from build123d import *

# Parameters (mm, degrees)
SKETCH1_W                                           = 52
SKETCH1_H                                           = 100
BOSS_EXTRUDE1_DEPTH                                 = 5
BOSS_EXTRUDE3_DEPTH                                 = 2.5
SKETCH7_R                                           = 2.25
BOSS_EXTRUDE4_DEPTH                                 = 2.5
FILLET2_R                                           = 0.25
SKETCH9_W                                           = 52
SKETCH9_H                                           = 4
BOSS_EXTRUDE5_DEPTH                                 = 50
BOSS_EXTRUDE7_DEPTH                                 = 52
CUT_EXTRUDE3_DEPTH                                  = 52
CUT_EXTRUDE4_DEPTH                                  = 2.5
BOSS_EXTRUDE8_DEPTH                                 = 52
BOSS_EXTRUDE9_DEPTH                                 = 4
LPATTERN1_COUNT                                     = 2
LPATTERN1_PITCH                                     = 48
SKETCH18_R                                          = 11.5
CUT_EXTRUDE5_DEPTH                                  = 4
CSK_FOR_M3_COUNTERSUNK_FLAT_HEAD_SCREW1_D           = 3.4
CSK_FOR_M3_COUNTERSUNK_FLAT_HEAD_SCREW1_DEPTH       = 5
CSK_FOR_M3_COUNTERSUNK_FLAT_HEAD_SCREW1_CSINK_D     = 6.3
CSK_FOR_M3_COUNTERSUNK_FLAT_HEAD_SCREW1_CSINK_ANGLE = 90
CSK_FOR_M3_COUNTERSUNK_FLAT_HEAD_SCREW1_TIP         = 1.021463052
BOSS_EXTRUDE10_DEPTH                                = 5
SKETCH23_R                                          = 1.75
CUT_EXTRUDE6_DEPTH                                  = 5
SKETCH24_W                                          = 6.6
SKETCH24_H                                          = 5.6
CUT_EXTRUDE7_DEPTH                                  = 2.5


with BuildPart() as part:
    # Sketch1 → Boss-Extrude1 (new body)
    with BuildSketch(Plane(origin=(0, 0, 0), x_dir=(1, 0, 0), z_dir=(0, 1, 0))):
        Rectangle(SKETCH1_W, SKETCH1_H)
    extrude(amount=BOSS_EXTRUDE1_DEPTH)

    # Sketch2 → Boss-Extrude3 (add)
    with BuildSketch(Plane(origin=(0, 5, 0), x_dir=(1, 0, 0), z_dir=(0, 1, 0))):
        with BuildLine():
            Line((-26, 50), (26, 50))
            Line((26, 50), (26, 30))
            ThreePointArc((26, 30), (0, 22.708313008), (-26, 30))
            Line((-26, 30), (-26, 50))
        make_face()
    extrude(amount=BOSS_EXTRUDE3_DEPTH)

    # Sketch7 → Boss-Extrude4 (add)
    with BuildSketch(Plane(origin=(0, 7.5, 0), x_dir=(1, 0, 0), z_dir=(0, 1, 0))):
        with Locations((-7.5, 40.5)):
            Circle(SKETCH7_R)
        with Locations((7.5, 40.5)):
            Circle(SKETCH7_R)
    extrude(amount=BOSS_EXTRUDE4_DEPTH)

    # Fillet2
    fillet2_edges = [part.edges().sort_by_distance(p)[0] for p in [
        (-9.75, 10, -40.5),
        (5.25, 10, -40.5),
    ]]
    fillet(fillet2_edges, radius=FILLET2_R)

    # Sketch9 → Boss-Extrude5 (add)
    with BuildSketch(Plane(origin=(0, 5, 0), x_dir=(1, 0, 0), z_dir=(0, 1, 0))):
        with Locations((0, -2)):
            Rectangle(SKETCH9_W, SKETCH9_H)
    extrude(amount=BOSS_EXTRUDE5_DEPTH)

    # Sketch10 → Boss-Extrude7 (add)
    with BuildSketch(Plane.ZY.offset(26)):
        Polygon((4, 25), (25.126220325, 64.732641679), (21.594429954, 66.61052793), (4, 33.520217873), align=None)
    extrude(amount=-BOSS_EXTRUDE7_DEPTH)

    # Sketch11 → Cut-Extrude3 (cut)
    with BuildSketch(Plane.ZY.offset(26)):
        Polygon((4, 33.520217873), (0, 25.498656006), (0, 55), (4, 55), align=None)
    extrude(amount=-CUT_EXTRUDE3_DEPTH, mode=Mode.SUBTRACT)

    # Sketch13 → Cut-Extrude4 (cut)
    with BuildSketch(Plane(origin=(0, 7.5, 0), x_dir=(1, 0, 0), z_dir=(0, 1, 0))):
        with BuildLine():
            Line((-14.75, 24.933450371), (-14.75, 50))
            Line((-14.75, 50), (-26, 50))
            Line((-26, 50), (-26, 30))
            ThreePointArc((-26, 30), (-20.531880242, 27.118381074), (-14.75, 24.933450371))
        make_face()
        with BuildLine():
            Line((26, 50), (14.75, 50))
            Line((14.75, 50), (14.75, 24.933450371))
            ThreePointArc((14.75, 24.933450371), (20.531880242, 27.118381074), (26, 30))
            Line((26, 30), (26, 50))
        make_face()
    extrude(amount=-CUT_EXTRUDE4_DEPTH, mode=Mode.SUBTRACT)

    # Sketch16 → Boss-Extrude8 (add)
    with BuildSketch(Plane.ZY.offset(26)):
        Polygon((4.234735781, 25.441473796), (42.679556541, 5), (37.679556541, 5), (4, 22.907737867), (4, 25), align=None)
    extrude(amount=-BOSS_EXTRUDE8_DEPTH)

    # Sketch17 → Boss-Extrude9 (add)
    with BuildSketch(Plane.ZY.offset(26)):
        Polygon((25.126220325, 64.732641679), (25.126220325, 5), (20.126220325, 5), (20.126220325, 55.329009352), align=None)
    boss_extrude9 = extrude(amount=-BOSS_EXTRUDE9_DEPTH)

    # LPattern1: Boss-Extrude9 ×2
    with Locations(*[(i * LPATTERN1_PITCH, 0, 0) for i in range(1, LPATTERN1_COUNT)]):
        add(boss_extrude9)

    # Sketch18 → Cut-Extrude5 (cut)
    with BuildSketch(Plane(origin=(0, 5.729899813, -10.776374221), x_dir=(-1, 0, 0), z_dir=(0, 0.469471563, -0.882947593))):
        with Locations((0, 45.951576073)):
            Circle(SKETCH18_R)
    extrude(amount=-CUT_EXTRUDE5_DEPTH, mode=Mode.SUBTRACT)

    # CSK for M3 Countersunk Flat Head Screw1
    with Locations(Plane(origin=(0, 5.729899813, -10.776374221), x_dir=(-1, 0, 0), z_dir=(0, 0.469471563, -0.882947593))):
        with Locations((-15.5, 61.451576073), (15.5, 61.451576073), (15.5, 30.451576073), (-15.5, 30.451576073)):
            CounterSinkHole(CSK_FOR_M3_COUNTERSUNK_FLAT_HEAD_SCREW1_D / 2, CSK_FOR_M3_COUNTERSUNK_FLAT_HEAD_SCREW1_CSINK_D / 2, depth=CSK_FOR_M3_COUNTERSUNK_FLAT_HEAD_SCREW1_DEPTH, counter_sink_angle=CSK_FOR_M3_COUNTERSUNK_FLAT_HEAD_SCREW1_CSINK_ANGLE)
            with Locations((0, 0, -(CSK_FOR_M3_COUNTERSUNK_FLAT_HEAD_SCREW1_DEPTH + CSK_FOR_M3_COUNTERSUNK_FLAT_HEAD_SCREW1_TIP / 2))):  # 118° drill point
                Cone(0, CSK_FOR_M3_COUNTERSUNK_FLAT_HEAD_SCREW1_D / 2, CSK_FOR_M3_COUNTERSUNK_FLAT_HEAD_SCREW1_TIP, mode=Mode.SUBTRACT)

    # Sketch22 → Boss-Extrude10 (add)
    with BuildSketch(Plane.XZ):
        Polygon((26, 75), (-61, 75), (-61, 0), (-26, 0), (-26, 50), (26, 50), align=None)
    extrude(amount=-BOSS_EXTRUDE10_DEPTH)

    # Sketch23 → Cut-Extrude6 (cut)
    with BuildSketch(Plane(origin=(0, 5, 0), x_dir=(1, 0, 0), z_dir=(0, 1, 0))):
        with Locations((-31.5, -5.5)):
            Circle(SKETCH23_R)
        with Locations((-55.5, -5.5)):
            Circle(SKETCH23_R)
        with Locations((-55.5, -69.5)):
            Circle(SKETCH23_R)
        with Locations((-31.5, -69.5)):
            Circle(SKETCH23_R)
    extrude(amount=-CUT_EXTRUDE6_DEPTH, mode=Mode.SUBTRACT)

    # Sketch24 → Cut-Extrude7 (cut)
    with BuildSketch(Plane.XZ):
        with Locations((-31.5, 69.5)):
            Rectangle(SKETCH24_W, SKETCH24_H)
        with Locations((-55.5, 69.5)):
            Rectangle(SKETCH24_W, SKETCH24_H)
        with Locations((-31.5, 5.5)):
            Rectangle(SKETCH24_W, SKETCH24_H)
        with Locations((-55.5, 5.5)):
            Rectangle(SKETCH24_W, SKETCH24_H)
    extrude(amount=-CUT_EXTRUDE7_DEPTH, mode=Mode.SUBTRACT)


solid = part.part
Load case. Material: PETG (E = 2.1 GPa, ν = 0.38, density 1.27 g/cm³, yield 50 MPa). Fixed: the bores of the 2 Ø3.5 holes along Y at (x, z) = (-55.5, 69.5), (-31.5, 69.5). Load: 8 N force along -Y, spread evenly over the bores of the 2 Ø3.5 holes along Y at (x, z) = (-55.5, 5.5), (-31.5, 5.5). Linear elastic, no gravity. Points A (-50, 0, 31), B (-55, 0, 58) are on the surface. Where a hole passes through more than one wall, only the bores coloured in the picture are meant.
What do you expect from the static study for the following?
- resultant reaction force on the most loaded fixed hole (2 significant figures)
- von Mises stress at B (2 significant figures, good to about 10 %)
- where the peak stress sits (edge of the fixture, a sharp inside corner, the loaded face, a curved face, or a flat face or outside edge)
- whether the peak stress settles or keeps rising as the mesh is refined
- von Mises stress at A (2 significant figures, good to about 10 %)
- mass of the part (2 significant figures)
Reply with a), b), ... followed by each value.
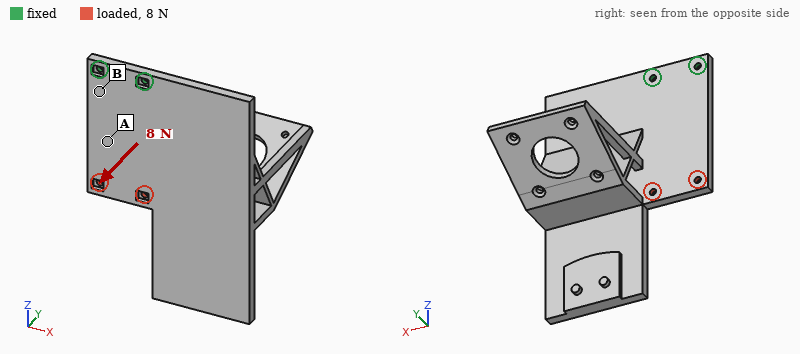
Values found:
a) 7.6 N
b) 1.9 MPa
c) edge of the fixture
d) keeps rising
e) 0.73 MPa
f) 84 g
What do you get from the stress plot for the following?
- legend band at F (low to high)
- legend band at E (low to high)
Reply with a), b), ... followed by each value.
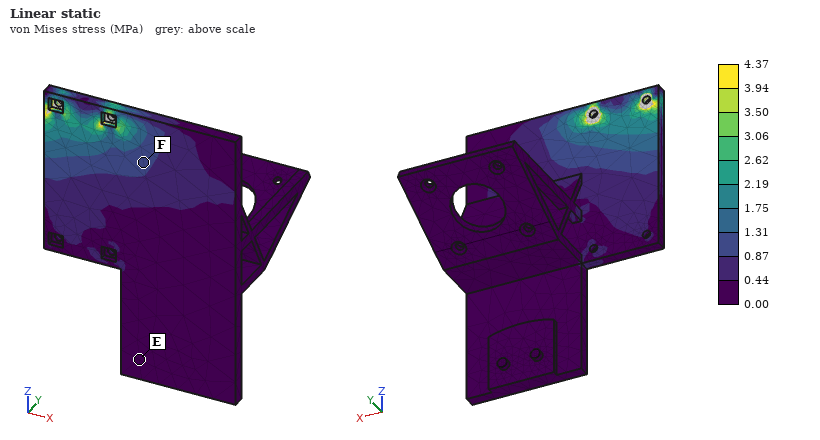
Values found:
a) 0.87 to 1.31 MPa
b) 0.00 to 0.44 MPa
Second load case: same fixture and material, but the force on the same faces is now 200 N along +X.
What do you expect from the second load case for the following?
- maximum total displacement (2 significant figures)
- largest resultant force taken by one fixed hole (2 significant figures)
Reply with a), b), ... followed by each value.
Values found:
a) 1.7 mm
b) 520 N
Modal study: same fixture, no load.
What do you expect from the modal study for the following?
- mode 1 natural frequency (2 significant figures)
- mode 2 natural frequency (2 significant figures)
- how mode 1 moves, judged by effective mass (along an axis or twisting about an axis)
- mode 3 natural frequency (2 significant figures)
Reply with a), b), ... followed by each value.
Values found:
a) 44 Hz
b) 130 Hz
c) along Y
d) 300 Hz
